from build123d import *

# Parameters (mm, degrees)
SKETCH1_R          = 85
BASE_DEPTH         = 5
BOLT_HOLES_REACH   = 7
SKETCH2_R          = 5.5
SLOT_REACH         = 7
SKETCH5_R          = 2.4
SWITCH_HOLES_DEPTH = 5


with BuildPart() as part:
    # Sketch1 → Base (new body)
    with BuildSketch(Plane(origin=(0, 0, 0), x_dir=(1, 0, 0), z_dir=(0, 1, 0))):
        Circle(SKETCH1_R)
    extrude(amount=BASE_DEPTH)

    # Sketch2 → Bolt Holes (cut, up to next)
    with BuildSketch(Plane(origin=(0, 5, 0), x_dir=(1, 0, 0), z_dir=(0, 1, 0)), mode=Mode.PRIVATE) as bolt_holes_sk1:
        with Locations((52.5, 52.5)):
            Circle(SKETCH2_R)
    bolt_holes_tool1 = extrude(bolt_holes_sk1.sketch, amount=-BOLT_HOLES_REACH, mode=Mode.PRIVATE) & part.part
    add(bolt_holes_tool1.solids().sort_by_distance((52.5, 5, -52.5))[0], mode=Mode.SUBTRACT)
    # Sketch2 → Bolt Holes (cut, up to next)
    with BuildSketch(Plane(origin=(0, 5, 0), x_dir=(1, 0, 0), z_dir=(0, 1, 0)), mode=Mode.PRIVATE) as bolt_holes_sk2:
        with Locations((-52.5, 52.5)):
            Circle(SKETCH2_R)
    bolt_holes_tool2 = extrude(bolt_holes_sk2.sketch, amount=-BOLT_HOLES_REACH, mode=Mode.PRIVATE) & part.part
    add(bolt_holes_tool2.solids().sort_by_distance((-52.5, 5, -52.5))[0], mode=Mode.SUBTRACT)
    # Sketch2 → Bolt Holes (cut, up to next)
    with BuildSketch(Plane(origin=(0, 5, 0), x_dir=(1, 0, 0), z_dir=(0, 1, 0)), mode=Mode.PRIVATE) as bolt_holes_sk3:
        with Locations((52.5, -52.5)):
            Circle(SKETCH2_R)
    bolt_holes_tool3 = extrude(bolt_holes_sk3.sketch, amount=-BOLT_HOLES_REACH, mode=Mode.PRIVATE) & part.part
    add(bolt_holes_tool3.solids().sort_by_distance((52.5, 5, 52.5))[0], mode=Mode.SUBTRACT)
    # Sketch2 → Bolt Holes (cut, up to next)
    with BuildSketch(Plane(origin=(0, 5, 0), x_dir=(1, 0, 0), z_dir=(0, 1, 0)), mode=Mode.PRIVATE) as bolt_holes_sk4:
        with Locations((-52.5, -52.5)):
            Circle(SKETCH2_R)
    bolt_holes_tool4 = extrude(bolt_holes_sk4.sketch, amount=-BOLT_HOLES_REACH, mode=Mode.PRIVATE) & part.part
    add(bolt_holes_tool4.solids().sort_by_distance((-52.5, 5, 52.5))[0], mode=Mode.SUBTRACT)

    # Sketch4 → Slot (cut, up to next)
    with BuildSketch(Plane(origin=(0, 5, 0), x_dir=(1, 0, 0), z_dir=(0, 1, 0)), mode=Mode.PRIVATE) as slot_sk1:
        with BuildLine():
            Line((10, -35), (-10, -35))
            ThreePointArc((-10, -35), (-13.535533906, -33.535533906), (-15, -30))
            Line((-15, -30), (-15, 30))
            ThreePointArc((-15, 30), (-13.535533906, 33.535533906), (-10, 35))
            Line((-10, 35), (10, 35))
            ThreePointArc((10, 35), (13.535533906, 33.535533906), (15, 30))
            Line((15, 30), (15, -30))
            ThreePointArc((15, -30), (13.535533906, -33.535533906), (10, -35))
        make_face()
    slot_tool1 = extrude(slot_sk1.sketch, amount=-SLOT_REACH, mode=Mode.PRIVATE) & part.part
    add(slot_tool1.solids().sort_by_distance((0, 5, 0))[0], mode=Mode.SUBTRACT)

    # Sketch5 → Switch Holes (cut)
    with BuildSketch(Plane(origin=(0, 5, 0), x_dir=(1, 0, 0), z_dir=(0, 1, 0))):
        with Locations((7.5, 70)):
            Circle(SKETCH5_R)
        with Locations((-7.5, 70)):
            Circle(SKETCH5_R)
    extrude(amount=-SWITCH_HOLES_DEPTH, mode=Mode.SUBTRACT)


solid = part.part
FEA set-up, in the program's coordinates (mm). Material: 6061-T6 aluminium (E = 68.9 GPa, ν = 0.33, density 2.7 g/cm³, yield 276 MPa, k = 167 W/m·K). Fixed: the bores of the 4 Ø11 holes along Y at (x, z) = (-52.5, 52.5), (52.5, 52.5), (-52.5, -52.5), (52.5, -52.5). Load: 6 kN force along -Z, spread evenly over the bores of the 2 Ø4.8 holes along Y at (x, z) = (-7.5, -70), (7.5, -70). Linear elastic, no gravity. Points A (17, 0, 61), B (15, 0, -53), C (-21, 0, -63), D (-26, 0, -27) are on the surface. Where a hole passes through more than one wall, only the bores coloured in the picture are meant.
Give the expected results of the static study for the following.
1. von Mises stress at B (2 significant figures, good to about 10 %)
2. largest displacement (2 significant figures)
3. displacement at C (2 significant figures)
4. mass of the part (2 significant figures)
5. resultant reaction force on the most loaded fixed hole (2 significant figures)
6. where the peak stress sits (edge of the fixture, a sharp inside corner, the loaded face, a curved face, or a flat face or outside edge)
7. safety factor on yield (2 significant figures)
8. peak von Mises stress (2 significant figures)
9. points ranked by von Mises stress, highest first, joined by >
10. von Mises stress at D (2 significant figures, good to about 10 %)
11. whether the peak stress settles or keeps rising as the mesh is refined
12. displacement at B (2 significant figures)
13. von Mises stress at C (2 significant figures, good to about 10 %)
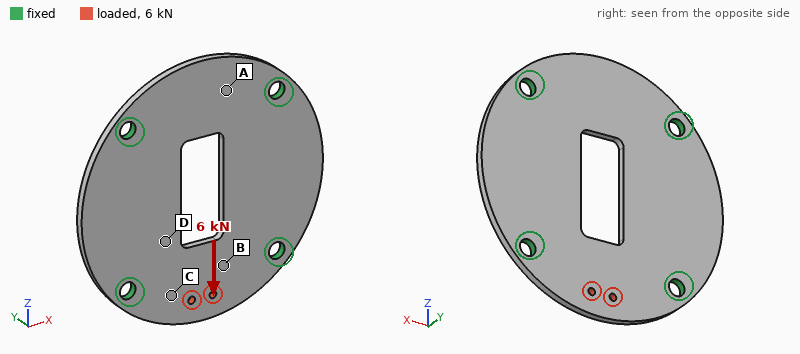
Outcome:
25 MPa
30 µm
17 µm
270 g
2.2 kN
the loaded face
3.6
77 MPa
B > C > D > A
14 MPa
settles
19 µm
21 MPa
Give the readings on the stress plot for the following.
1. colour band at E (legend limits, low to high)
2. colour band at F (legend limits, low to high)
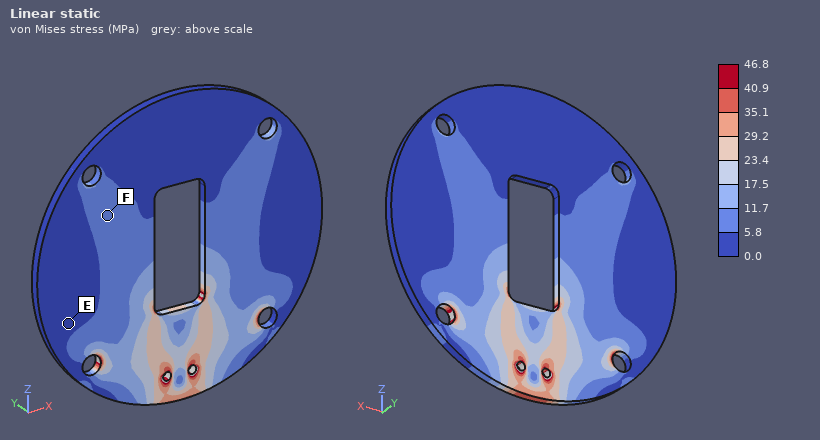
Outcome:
0.0 to 5.8 MPa
5.8 to 11.7 MPa
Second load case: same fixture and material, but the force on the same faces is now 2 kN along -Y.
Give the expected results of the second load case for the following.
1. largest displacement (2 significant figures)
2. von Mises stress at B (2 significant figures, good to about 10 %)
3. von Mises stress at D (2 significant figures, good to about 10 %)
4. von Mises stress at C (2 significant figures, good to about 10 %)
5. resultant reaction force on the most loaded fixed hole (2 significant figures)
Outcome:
0.69 mm
74 MPa
35 MPa
61 MPa
1.1 kN
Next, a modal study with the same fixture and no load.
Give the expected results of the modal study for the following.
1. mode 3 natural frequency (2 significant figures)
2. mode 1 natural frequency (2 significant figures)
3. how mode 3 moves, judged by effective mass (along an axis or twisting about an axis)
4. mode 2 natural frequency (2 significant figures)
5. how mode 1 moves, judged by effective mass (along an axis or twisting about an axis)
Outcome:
2200 Hz
2000 Hz
twisting about Z
2100 Hz
along Y
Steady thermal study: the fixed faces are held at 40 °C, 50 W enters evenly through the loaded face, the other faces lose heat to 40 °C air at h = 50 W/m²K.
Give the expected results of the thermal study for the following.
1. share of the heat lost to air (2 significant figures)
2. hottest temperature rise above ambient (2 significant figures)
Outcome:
21 %
37 K
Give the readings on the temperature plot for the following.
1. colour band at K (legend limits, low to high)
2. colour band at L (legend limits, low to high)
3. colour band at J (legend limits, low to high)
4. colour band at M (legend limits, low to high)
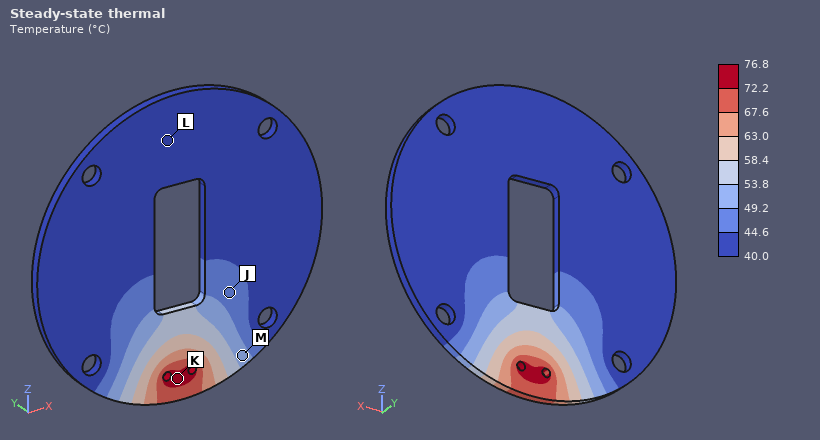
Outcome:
72.2 to 76.8 °C
40.0 to 44.6 °C
44.6 to 49.2 °C
49.2 to 53.8 °C
